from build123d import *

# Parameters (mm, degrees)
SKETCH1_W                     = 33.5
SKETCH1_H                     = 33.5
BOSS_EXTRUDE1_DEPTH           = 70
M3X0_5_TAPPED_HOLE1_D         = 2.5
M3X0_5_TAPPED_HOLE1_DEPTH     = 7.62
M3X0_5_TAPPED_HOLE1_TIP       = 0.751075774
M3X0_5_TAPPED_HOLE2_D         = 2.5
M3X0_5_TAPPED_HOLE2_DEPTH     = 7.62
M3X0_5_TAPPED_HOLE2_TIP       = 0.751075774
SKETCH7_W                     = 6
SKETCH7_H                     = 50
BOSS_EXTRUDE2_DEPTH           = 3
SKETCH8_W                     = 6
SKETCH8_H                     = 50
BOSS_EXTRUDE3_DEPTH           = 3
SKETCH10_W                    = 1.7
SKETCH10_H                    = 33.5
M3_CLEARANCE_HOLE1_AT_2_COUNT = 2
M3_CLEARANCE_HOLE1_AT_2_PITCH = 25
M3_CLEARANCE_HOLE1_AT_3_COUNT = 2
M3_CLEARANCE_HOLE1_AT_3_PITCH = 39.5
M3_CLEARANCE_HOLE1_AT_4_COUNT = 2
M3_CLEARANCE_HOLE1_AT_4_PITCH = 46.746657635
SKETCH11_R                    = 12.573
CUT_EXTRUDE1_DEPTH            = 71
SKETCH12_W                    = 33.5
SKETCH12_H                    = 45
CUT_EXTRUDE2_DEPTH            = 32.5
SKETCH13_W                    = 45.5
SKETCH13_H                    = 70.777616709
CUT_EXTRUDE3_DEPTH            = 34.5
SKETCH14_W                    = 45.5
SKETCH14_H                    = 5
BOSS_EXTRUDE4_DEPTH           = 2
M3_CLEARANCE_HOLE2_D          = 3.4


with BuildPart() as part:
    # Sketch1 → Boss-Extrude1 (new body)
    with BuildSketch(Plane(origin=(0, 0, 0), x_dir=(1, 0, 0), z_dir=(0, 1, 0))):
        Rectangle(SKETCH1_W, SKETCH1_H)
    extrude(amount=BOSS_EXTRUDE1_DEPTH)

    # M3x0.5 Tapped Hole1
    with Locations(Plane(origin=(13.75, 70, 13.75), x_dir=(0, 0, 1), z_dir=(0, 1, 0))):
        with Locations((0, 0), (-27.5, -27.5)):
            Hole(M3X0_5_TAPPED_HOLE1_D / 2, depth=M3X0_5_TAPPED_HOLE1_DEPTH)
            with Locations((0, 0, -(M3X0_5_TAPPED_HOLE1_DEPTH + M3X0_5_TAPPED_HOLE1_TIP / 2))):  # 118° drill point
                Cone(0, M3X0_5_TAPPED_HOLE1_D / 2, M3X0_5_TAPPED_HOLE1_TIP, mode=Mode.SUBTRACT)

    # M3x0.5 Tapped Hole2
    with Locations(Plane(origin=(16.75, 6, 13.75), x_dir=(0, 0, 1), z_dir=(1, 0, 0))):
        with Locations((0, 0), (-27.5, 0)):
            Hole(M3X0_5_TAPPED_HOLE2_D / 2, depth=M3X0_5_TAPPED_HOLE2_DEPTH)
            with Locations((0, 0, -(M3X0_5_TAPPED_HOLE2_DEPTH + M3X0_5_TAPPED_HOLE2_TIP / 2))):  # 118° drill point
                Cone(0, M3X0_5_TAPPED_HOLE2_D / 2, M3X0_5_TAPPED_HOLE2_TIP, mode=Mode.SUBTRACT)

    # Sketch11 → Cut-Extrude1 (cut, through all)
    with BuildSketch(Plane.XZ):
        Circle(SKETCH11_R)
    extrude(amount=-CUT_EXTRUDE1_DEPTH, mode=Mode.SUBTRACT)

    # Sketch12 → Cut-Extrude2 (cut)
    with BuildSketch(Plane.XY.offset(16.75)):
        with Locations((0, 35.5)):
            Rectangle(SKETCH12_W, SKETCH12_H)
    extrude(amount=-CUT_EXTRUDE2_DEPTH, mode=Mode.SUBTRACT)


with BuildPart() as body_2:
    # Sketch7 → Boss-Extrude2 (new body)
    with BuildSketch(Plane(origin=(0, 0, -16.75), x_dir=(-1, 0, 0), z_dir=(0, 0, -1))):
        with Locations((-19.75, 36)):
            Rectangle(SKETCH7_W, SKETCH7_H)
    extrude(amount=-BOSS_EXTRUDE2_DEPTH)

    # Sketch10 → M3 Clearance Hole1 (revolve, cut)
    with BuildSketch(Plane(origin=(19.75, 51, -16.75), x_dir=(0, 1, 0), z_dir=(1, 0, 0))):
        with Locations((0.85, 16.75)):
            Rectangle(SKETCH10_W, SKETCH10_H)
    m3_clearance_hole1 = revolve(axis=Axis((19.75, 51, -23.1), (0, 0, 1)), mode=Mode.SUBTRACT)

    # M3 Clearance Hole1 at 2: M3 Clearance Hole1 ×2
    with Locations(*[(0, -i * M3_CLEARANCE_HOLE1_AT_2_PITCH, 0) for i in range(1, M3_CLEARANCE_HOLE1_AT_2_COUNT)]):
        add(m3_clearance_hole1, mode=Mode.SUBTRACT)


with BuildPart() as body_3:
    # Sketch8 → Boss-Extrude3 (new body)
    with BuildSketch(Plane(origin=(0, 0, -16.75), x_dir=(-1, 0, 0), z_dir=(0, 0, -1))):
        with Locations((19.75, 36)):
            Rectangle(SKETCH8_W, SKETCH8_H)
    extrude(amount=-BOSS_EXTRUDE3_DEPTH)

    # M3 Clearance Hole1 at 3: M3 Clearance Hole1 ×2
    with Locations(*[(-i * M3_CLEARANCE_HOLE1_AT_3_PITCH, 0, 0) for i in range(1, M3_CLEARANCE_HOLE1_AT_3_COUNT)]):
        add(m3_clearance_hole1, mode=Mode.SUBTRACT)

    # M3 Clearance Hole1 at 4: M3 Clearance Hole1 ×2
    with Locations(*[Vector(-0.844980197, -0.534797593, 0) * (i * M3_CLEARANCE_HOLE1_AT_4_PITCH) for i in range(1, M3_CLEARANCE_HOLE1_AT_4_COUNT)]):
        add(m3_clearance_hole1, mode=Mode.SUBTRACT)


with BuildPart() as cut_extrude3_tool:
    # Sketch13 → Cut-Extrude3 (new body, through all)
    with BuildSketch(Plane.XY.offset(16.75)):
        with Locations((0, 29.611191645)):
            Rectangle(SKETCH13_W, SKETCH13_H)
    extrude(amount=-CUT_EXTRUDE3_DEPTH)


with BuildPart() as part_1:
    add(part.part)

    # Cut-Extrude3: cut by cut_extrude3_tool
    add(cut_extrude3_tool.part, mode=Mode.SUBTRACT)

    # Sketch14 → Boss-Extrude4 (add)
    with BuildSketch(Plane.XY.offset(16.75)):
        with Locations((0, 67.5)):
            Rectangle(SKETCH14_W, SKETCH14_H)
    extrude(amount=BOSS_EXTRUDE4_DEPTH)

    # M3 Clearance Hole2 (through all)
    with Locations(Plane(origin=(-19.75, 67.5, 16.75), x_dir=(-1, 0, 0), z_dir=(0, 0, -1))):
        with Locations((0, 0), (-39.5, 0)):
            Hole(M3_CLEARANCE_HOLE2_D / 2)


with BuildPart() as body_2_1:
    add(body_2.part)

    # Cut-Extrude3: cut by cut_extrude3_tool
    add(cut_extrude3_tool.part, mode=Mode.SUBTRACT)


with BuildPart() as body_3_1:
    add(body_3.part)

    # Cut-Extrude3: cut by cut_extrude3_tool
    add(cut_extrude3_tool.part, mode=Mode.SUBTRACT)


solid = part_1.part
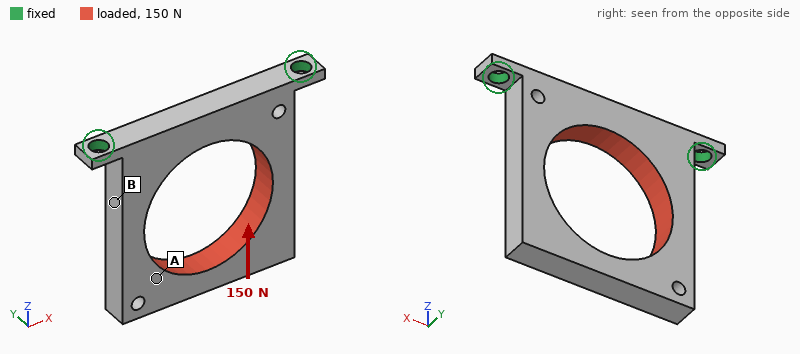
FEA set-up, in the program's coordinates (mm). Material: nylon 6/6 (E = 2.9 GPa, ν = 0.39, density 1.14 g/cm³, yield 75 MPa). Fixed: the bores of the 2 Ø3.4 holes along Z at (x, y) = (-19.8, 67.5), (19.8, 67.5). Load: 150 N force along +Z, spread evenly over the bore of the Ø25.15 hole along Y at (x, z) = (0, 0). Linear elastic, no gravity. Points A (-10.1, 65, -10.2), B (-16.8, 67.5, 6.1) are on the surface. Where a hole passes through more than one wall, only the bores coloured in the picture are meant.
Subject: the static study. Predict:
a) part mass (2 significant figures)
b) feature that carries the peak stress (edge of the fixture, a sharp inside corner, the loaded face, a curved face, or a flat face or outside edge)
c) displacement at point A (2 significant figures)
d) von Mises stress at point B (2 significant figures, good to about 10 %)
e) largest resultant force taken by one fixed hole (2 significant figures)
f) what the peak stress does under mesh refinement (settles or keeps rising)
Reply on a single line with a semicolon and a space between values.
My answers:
4.0 g; edge of the fixture; 60 µm; 4.8 MPa; 86 N; keeps rising
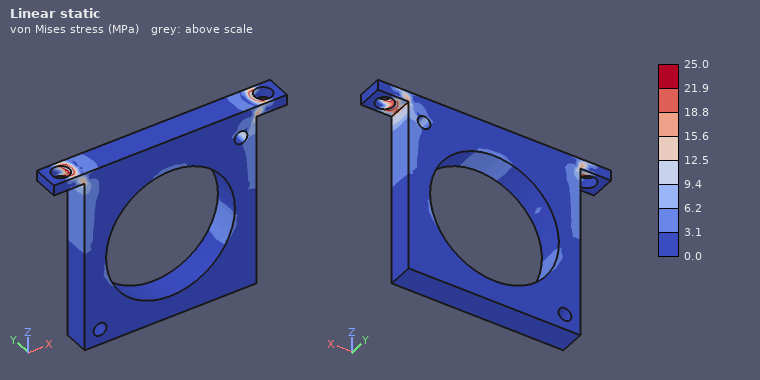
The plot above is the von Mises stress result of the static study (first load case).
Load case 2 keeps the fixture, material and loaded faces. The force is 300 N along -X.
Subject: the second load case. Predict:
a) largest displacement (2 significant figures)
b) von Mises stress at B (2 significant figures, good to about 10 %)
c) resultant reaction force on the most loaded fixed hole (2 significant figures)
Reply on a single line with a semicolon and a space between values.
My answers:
0.67 mm; 20 MPa; 220 N
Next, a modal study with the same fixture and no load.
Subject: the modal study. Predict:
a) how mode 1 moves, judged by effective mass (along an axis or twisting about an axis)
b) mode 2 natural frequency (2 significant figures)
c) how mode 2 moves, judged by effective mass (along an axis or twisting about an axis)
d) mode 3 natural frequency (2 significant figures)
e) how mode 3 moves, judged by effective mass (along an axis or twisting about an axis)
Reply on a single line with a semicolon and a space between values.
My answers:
along Y; 1400 Hz; twisting about Z; 2000 Hz; along X
